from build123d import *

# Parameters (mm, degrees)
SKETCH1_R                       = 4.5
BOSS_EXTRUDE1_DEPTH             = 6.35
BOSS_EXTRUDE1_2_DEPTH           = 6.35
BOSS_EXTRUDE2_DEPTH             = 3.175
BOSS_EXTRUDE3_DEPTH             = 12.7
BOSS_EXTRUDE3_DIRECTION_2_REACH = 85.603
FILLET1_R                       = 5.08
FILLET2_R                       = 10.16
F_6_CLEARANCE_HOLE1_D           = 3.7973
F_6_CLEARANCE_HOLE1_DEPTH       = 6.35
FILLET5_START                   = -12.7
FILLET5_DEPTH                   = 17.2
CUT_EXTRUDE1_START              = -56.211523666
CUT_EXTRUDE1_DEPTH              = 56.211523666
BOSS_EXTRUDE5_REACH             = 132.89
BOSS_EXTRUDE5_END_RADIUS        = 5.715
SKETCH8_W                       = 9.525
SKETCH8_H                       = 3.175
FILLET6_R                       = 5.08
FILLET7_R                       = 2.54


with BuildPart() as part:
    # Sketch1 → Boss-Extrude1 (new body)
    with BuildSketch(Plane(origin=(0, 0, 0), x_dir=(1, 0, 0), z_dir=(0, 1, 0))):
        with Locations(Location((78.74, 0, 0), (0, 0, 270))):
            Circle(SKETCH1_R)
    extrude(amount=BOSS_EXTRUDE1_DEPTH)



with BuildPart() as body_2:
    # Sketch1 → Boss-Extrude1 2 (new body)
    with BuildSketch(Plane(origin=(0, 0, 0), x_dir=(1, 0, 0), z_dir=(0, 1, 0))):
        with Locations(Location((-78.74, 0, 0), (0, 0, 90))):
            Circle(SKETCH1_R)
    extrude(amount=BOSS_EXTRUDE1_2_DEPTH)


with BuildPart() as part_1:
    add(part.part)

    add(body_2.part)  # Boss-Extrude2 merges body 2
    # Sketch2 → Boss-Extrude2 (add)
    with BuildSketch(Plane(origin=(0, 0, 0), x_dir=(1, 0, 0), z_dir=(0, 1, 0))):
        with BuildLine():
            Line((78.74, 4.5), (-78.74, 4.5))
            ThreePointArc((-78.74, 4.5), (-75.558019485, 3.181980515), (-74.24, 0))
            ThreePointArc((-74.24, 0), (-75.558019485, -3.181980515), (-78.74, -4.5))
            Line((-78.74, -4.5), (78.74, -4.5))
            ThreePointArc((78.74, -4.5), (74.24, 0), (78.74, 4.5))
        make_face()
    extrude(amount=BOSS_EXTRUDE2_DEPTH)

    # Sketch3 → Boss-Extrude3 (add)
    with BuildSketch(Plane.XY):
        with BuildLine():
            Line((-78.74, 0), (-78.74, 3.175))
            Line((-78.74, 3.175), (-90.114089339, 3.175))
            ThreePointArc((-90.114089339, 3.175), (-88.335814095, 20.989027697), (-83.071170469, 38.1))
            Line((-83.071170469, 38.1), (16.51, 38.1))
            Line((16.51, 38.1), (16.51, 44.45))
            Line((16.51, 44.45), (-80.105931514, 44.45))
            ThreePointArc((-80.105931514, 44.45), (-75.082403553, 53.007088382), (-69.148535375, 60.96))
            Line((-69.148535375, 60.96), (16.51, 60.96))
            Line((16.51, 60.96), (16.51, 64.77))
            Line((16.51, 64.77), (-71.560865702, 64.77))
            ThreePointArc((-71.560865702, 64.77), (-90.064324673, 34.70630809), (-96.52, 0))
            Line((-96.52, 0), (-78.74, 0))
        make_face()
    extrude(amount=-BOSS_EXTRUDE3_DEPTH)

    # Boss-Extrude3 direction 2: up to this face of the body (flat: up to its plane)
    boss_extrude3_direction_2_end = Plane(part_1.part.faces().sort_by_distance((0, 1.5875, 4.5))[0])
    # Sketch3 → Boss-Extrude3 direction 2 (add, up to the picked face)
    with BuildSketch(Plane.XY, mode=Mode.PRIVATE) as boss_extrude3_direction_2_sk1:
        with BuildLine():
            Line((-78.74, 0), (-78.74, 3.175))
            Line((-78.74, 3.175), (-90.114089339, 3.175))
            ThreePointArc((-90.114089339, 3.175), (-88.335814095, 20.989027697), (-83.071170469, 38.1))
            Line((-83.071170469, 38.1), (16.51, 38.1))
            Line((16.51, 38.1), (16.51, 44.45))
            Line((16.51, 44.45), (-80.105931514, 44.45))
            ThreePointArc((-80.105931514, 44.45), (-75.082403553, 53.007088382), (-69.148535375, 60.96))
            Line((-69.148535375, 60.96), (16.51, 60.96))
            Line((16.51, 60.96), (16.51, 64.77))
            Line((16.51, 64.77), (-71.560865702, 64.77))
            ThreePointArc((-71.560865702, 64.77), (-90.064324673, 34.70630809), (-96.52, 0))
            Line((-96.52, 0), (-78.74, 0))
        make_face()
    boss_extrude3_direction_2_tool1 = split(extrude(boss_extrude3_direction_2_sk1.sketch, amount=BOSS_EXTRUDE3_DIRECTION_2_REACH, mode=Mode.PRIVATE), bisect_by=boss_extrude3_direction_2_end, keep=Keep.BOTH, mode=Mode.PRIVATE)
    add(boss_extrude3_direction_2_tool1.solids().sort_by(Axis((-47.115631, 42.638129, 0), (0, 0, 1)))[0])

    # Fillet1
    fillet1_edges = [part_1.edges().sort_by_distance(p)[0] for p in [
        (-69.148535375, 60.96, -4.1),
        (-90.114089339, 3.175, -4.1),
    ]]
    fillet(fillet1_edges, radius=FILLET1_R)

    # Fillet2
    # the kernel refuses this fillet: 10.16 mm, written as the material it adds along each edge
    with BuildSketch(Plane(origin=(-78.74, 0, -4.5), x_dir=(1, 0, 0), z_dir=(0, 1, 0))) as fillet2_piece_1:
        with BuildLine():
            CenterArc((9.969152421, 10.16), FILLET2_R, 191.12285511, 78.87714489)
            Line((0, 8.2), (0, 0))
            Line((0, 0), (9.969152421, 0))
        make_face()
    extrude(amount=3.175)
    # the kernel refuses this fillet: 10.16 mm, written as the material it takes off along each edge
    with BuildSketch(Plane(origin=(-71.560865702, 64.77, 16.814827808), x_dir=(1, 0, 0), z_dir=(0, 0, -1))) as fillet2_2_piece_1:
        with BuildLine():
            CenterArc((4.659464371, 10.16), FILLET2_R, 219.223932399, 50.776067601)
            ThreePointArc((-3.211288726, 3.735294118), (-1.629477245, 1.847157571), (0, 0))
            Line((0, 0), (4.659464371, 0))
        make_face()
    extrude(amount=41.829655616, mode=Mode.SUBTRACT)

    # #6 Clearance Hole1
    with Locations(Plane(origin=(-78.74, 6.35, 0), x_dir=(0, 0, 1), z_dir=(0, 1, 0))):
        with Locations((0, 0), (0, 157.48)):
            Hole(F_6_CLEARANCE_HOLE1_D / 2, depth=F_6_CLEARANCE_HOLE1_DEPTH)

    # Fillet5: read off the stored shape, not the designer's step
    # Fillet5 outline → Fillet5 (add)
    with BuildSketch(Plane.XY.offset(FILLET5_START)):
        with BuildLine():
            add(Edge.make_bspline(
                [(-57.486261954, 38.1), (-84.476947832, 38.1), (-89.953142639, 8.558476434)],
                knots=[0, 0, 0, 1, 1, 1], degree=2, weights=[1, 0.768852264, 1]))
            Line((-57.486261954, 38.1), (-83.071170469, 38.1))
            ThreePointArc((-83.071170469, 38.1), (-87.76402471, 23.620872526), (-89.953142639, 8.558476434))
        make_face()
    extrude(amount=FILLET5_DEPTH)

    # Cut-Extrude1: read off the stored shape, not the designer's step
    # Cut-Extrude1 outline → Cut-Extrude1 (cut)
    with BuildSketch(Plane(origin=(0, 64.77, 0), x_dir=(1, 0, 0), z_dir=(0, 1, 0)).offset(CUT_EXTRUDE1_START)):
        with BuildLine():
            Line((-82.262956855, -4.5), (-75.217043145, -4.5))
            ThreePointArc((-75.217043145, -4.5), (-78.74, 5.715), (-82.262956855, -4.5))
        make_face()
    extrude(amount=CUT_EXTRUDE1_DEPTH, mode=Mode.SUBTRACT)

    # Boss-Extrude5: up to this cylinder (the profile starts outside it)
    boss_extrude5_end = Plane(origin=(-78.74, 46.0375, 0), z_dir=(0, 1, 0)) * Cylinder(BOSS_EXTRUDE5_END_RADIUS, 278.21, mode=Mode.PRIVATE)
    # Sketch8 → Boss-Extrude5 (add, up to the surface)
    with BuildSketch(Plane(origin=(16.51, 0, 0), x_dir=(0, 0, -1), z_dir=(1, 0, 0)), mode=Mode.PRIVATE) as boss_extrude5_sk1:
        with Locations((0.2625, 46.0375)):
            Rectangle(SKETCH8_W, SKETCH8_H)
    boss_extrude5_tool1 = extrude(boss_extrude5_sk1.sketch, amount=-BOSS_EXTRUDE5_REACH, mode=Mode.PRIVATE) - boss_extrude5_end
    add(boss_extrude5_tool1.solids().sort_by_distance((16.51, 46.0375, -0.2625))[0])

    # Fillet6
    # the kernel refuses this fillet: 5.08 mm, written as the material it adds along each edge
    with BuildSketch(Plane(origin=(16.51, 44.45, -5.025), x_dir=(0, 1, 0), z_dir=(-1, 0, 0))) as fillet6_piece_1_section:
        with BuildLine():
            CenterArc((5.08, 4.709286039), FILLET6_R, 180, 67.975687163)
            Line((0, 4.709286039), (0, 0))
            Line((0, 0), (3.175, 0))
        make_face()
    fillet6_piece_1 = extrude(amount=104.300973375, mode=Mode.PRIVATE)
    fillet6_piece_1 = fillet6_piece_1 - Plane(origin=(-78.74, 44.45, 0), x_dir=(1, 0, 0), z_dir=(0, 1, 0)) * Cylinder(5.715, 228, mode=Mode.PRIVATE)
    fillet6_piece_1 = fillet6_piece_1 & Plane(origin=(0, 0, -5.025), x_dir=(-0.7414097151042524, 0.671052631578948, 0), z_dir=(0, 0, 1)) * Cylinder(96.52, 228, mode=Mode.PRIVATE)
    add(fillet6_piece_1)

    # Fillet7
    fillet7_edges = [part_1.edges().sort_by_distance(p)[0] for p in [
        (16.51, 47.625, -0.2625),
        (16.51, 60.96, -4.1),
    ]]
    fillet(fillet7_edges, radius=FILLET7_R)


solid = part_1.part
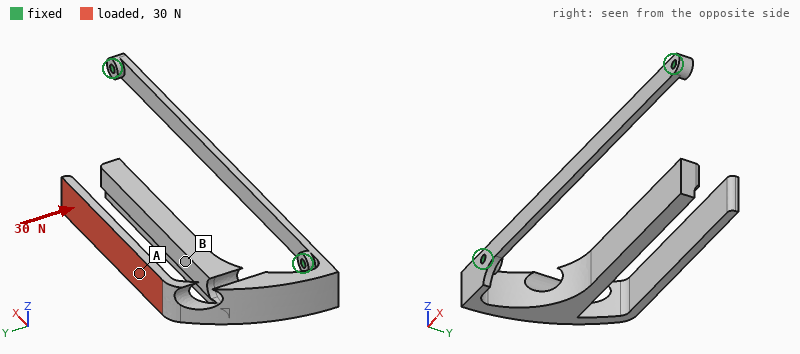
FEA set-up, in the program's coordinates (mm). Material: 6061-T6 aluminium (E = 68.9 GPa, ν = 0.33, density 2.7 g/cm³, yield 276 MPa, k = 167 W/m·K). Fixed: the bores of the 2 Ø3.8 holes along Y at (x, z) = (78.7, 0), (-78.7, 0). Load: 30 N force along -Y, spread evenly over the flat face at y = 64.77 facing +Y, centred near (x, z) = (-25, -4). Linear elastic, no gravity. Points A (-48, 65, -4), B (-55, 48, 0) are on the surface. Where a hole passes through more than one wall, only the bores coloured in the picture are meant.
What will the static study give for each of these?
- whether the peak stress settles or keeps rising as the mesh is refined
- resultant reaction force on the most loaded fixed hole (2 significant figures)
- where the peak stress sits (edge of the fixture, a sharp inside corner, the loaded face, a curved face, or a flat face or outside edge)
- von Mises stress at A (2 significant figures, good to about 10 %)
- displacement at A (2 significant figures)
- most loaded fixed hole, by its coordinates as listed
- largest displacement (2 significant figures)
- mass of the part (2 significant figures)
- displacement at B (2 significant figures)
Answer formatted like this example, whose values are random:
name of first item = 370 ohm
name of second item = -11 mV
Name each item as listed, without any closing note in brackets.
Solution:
whether the peak stress settles or keeps rising as the mesh is refined = keeps rising
resultant reaction force on the most loaded fixed hole = 30 N
where the peak stress sits = a sharp inside corner
von Mises stress at A = 18 MPa
displacement at A = 0.71 mm
most loaded fixed hole, by its coordinates as listed = (-78.7, 0)
largest displacement = 1.9 mm
mass of the part = 87 g
displacement at B = 0.33 mm
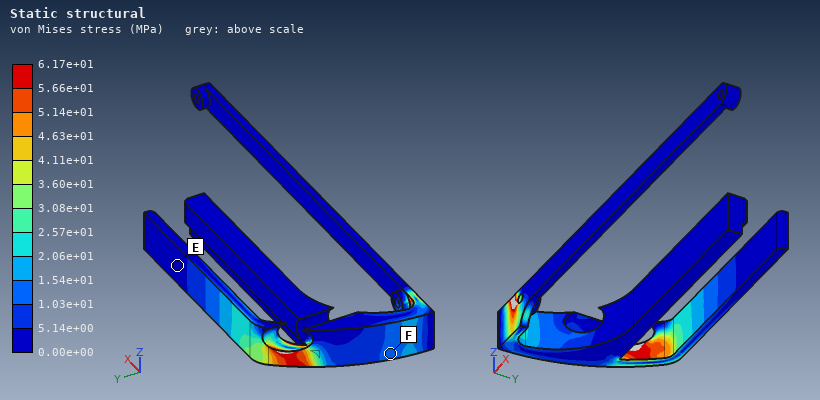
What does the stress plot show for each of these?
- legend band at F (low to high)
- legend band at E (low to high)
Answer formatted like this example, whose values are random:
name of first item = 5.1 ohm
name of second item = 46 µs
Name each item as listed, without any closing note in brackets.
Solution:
legend band at F = 1.03e+01 to 1.54e+01 MPa
legend band at E = 0.00e+00 to 5.14e+00 MPa
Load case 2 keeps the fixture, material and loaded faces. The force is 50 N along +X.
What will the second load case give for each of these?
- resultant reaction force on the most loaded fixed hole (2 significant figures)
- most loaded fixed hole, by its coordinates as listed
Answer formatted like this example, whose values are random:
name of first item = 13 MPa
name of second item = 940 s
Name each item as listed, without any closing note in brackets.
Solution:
resultant reaction force on the most loaded fixed hole = 51 N
most loaded fixed hole, by its coordinates as listed = (-78.7, 0)
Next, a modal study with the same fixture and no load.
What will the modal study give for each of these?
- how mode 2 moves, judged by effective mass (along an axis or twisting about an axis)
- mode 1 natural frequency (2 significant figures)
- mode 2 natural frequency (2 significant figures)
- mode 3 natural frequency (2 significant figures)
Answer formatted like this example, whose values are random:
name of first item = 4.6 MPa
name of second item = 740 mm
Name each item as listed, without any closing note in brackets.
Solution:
how mode 2 moves, judged by effective mass = along Z
mode 1 natural frequency = 140 Hz
mode 2 natural frequency = 220 Hz
mode 3 natural frequency = 300 Hz
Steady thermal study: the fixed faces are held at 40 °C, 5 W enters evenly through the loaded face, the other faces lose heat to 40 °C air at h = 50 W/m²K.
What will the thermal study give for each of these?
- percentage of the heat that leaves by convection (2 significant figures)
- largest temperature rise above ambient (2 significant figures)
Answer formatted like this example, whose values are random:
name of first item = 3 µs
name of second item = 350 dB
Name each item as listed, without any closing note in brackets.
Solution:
percentage of the heat that leaves by convection = 76 %
largest temperature rise above ambient = 24 K
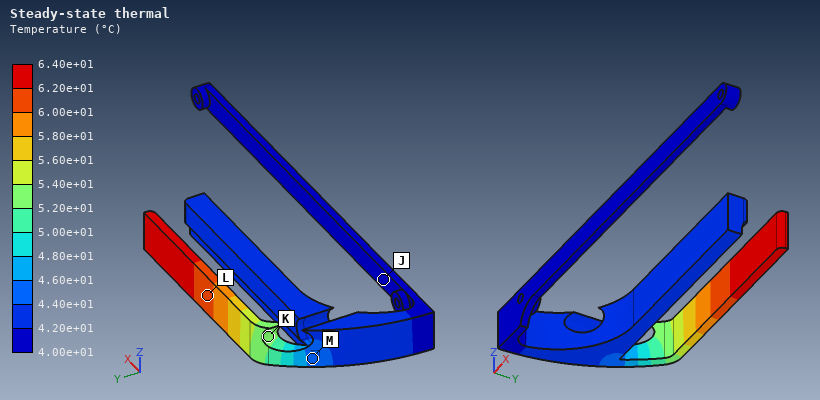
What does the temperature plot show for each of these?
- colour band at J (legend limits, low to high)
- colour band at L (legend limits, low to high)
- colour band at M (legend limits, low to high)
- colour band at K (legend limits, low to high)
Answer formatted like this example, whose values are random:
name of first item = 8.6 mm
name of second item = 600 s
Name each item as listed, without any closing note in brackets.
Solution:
colour band at J = 4.00e+01 to 4.20e+01 °C
colour band at L = 6.00e+01 to 6.20e+01 °C
colour band at M = 4.40e+01 to 4.60e+01 °C
colour band at K = 5.20e+01 to 5.40e+01 °C
